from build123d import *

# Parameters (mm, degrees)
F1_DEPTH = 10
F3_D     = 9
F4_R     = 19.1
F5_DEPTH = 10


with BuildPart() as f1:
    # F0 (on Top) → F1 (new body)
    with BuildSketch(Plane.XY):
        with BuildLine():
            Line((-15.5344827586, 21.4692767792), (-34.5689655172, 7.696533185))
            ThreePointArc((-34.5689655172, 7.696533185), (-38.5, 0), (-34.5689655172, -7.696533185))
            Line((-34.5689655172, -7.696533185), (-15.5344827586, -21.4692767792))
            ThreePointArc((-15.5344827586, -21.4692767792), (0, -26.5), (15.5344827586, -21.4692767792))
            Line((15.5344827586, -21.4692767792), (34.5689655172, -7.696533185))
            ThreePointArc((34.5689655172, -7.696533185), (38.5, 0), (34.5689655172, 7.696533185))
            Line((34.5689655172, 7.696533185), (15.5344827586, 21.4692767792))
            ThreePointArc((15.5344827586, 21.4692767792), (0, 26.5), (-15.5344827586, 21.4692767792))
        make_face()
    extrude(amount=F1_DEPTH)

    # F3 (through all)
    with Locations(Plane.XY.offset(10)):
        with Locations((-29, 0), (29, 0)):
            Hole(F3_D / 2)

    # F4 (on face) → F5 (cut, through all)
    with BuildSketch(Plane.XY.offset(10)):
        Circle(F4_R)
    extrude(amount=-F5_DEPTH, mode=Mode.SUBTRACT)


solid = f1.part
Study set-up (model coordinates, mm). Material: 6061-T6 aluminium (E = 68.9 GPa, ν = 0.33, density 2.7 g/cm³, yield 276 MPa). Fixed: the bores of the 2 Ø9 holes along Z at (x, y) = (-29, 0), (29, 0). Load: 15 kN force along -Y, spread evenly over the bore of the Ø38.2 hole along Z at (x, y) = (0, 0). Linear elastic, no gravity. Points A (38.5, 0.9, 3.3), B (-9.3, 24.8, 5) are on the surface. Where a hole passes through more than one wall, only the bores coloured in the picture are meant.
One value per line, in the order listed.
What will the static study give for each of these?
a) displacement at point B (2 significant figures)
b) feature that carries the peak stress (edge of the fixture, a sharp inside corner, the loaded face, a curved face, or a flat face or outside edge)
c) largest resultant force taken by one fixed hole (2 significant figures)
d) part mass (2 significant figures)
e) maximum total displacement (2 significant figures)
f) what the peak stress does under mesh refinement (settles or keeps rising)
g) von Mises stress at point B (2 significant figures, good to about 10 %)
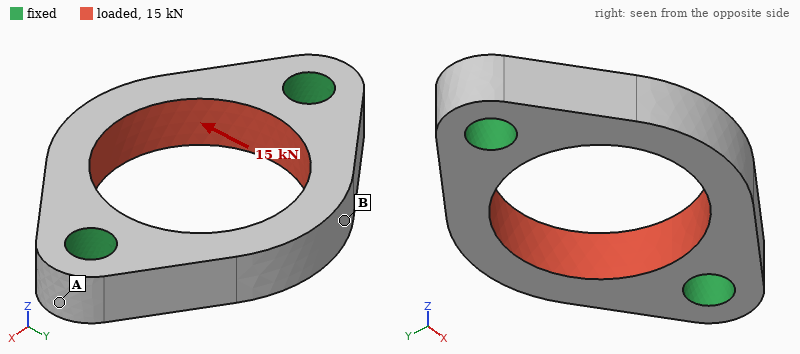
24 µm
edge of the fixture
7.5 kN
40 g
30 µm
keeps rising
42 MPa
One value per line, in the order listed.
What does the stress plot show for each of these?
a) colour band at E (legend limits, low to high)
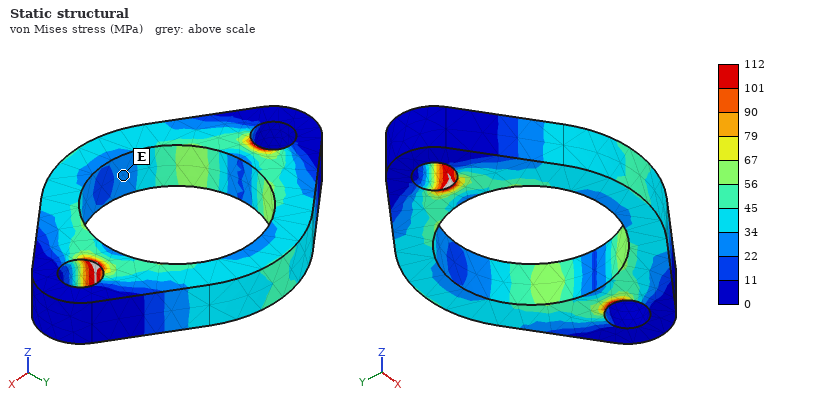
22 to 34 MPa
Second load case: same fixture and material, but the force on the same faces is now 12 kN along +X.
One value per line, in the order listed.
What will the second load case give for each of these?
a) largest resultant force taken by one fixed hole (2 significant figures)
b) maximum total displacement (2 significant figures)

6.0 kN
26 µm
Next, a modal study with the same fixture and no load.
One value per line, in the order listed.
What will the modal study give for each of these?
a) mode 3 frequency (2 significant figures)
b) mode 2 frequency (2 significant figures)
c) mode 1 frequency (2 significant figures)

19 kHz
9400 Hz
9100 Hz
